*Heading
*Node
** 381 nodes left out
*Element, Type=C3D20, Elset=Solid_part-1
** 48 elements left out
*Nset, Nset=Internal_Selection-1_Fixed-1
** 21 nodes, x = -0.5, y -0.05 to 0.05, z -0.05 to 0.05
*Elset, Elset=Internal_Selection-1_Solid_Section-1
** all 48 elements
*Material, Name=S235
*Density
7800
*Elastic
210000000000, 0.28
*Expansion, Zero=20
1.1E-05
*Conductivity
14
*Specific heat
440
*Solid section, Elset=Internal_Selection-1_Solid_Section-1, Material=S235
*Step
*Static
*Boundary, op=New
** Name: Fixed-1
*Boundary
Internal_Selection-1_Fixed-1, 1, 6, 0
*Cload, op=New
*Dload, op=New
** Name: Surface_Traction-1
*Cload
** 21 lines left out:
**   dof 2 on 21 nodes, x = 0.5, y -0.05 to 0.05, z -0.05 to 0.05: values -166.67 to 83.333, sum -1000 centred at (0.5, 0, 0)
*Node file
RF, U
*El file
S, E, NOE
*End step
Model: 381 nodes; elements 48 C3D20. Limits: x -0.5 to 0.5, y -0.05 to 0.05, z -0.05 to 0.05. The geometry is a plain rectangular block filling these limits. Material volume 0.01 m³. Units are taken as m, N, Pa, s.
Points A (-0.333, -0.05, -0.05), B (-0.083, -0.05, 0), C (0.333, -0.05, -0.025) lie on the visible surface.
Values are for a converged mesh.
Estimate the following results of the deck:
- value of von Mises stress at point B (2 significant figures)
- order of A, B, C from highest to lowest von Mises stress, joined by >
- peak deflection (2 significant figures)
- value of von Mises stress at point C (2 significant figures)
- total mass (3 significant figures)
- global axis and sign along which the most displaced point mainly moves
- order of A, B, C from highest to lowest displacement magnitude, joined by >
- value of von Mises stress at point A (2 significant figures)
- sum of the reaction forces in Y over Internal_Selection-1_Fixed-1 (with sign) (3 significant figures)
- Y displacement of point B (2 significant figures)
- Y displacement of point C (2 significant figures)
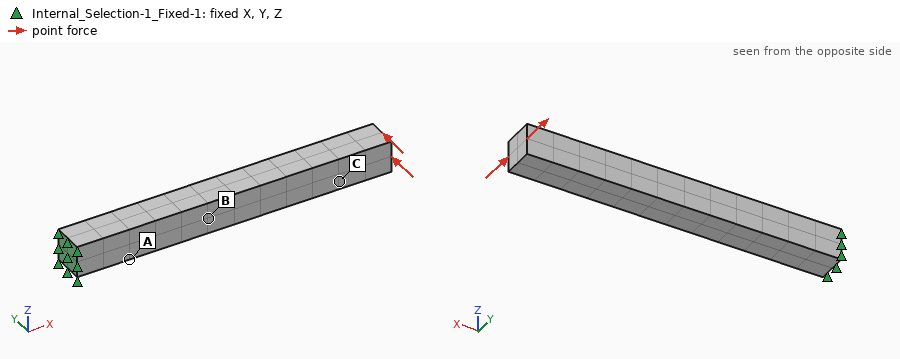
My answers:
3.5e+06 Pa
A > B > C
1.9e-04 m
1.0e+06 Pa
78.0 kg
-Y
C > B > A
5.0e+06 Pa
1000 N
-4.3e-05 m
-1.4e-04 m
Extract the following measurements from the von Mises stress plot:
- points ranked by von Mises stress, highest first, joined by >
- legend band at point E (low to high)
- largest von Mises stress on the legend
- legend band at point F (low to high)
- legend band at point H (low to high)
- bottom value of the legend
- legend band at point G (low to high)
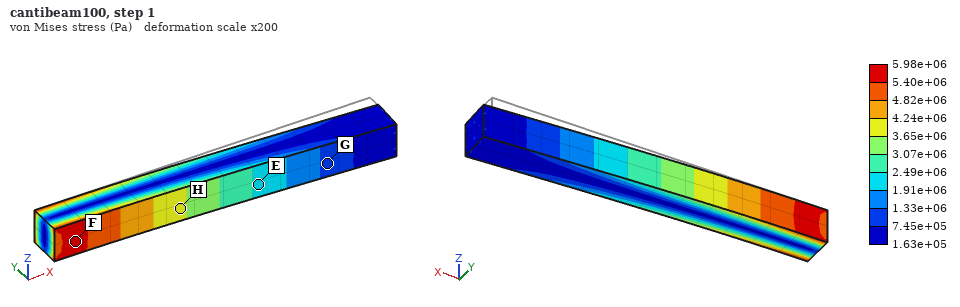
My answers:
F > H > E > G
1.91e+06 to 2.49e+06 Pa
5.98e+06 Pa
5.40e+06 to 5.98e+06 Pa
3.65e+06 to 4.24e+06 Pa
1.63e+05 Pa
7.45e+05 to 1.33e+06 Pa
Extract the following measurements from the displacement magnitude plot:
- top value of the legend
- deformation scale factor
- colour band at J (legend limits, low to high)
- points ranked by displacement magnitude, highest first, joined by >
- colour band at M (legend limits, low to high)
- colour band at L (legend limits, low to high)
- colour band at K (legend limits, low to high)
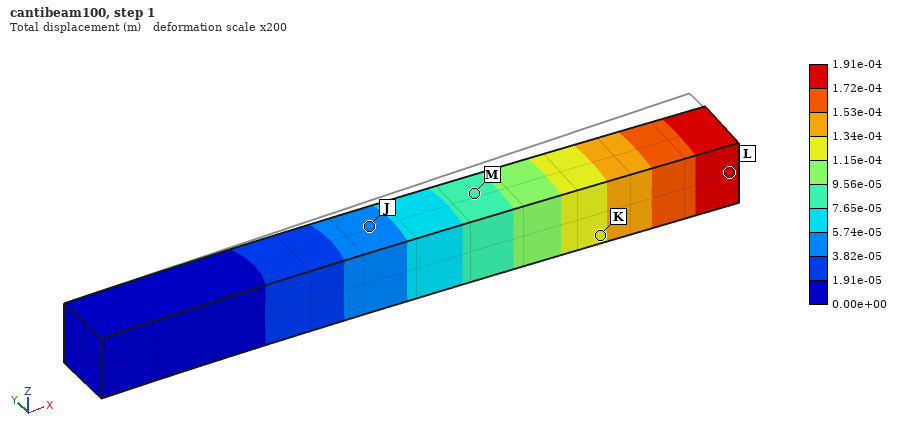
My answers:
1.91e-04 m
200
3.82e-05 to 5.74e-05 m
L > K > M > J
7.65e-05 to 9.56e-05 m
1.72e-04 to 1.91e-04 m
1.15e-04 to 1.34e-04 m
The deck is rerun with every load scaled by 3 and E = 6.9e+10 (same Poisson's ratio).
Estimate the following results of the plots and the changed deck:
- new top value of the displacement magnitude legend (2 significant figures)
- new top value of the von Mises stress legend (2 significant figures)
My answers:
0.0017 m
1.8e+07 Pa
